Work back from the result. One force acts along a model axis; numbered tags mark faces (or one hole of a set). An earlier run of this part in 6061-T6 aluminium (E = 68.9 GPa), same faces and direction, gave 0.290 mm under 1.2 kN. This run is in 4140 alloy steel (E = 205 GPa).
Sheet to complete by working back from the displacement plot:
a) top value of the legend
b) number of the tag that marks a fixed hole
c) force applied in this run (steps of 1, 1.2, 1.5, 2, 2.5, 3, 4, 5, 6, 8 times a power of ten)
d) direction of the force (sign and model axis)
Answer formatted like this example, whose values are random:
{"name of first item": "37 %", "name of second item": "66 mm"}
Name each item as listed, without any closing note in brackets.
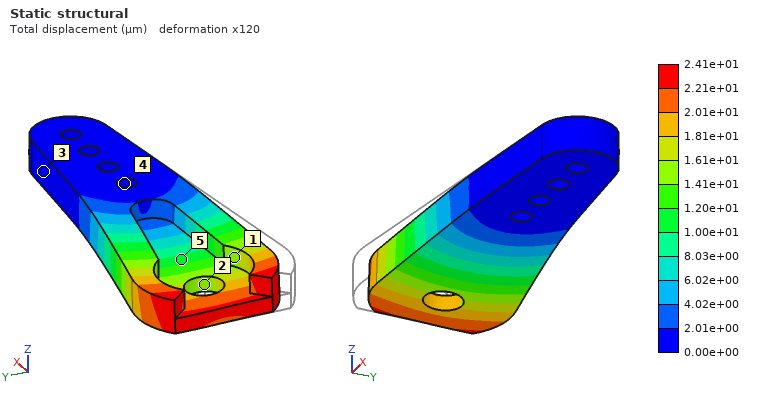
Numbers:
{"top value of the legend": "2.41e+01 µm", "number of the tag that marks a fixed hole": "4", "force applied in this run": "300 N", "direction of the force": "+Y"}
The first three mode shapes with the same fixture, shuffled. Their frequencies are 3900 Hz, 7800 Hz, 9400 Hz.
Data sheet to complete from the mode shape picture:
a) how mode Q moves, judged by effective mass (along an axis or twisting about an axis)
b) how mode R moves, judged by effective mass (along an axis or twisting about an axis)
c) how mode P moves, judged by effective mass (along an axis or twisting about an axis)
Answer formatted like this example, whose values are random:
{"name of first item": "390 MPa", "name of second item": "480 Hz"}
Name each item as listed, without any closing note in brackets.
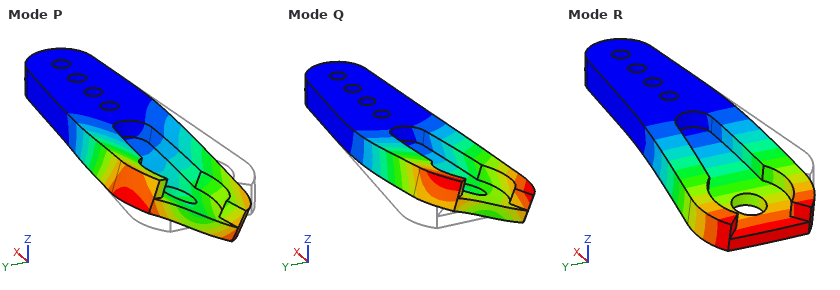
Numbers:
{"how mode Q moves, judged by effective mass": "along Y", "how mode R moves, judged by effective mass": "along Z", "how mode P moves, judged by effective mass": "along Y"}
